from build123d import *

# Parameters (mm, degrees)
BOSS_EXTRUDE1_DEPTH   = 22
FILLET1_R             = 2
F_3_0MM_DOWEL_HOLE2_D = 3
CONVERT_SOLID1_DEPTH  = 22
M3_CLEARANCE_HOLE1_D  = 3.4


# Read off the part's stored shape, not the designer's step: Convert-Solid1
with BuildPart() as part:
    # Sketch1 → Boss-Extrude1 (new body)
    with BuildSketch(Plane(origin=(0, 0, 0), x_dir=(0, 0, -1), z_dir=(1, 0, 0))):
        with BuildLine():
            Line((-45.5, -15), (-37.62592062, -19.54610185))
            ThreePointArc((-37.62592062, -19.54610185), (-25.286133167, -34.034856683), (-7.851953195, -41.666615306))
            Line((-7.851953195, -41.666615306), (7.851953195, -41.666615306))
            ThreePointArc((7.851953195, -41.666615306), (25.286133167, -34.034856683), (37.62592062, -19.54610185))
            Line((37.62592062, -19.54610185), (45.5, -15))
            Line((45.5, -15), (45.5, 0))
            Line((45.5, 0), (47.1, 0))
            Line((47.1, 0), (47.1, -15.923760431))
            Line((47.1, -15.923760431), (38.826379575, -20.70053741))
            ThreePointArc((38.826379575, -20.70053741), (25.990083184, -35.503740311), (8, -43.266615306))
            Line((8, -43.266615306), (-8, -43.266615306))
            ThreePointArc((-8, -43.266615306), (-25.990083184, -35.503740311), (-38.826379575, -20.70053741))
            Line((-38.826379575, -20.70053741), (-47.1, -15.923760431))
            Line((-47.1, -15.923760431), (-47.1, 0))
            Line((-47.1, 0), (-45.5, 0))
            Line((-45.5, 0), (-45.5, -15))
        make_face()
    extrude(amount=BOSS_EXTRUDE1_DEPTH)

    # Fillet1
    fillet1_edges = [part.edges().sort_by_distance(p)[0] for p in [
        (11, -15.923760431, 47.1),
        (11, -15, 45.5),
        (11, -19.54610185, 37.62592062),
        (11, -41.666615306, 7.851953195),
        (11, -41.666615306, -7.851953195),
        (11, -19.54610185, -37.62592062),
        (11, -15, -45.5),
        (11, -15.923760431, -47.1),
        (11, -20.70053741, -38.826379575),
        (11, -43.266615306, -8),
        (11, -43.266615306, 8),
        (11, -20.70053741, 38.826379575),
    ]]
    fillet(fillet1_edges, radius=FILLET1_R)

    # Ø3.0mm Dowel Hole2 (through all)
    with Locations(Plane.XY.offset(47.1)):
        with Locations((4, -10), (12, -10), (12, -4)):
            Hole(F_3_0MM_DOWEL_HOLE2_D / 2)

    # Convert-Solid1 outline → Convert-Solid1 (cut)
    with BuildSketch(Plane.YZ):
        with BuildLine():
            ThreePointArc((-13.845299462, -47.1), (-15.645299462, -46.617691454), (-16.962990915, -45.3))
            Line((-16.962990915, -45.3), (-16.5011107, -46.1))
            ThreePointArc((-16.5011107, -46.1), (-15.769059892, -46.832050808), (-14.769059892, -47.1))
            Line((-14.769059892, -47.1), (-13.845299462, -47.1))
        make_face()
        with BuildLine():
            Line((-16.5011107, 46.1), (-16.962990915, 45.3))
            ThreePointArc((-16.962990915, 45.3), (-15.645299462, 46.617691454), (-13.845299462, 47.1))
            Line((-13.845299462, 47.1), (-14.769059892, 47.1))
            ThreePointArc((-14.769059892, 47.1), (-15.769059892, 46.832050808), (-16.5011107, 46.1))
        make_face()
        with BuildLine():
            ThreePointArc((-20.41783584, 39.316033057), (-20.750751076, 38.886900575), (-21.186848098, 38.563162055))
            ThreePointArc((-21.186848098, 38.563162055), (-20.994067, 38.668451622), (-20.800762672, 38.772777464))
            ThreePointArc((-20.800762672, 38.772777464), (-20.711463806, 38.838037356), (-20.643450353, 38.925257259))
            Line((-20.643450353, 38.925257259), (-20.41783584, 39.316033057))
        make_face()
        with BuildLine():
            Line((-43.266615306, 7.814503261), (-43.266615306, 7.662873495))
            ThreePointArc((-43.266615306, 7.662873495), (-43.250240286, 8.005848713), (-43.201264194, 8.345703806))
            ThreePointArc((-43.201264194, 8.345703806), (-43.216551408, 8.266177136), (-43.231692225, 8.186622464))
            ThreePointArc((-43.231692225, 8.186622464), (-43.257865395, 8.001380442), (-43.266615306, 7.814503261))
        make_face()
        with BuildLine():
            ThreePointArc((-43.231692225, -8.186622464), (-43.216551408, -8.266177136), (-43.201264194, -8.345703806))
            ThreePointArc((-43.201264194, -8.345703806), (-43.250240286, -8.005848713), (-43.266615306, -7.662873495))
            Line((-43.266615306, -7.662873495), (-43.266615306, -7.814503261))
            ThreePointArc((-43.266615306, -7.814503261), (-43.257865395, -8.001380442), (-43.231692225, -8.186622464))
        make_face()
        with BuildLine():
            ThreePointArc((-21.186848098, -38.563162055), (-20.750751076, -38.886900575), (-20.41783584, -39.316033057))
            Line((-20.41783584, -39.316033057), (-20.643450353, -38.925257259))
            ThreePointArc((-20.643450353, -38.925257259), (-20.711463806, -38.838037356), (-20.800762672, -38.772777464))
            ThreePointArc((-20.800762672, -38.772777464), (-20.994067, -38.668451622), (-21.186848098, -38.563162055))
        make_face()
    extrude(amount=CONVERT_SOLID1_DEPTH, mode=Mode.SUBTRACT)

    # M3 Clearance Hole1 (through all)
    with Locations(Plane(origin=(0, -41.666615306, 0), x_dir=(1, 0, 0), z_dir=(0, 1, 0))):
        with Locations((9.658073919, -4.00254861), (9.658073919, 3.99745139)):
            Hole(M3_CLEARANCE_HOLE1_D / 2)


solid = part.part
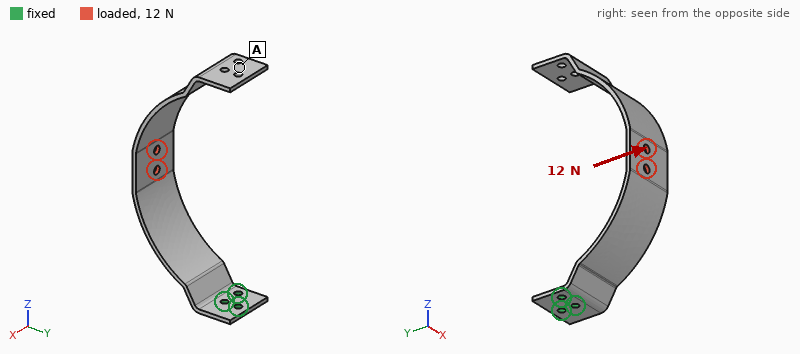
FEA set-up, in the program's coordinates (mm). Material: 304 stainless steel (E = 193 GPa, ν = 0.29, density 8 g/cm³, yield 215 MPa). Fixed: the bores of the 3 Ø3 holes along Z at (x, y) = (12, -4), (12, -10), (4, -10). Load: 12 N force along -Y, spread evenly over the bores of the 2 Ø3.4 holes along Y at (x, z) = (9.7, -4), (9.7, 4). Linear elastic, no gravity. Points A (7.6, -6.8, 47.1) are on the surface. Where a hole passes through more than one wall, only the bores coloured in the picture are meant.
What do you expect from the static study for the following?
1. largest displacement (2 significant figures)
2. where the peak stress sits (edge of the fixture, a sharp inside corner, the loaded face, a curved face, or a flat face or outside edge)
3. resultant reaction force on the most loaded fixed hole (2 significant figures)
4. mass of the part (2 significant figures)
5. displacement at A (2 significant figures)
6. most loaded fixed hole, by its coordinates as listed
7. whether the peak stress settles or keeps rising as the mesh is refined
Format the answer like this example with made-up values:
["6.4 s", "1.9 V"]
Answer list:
["1.1 mm", "edge of the fixture", "22 N", "39 g", "1.1 mm", "(12, -10)", "keeps rising"]
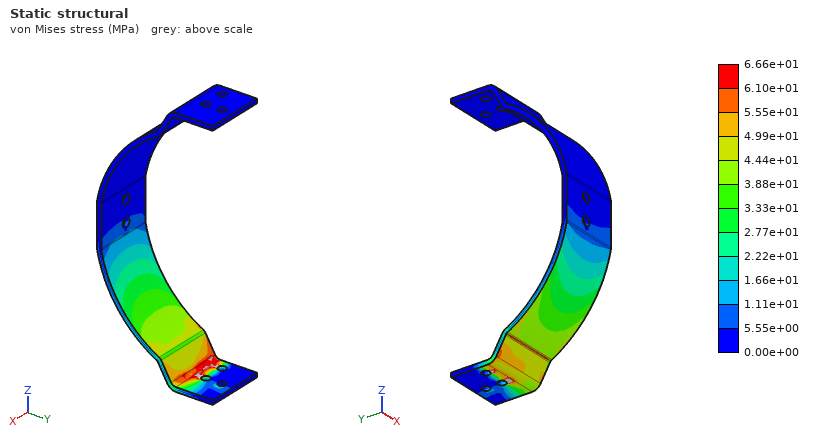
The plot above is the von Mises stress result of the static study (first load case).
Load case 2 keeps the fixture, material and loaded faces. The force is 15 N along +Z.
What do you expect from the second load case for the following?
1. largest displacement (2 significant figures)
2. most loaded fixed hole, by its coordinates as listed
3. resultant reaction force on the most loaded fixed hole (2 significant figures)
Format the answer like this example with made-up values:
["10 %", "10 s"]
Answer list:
["0.62 mm", "(12, -10)", "25 N"]
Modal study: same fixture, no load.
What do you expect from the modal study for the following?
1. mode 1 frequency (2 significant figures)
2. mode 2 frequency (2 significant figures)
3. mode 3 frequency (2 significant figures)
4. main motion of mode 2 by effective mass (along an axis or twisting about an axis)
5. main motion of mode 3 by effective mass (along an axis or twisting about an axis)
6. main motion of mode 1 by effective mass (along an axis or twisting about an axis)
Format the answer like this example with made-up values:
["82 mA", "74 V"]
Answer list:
["88 Hz", "160 Hz", "310 Hz", "along X", "along Z", "along Y"]
